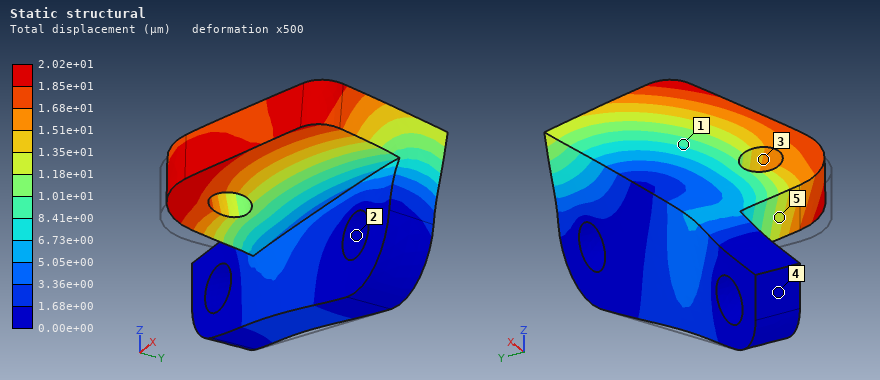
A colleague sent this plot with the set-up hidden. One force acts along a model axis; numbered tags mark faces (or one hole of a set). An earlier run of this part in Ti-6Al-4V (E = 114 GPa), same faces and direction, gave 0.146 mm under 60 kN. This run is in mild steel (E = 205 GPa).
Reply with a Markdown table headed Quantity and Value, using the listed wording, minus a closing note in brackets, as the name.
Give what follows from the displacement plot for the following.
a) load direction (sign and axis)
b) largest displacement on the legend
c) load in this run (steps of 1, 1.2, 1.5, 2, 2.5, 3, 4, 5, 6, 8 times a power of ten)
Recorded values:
| Quantity | Value |
|---|---|
| load direction | +X |
| largest displacement on the legend | 2.02e+01 µm |
| load in this run | 15 kN |
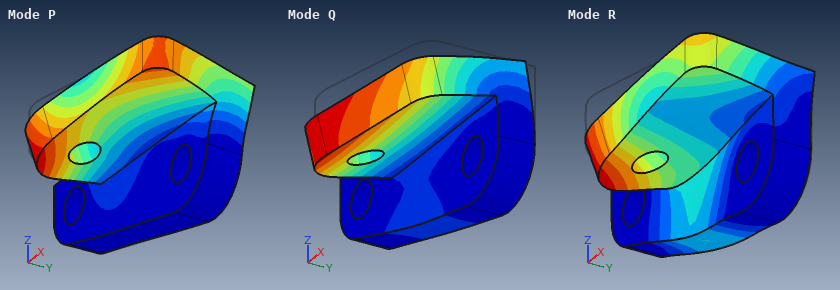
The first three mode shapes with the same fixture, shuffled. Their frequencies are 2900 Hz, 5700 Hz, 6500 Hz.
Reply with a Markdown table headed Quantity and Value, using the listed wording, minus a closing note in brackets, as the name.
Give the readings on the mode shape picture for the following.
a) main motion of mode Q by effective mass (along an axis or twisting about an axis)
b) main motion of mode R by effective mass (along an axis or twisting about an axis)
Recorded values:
| Quantity | Value |
|---|---|
| main motion of mode Q by effective mass | along Z |
| main motion of mode R by effective mass | along Y |
